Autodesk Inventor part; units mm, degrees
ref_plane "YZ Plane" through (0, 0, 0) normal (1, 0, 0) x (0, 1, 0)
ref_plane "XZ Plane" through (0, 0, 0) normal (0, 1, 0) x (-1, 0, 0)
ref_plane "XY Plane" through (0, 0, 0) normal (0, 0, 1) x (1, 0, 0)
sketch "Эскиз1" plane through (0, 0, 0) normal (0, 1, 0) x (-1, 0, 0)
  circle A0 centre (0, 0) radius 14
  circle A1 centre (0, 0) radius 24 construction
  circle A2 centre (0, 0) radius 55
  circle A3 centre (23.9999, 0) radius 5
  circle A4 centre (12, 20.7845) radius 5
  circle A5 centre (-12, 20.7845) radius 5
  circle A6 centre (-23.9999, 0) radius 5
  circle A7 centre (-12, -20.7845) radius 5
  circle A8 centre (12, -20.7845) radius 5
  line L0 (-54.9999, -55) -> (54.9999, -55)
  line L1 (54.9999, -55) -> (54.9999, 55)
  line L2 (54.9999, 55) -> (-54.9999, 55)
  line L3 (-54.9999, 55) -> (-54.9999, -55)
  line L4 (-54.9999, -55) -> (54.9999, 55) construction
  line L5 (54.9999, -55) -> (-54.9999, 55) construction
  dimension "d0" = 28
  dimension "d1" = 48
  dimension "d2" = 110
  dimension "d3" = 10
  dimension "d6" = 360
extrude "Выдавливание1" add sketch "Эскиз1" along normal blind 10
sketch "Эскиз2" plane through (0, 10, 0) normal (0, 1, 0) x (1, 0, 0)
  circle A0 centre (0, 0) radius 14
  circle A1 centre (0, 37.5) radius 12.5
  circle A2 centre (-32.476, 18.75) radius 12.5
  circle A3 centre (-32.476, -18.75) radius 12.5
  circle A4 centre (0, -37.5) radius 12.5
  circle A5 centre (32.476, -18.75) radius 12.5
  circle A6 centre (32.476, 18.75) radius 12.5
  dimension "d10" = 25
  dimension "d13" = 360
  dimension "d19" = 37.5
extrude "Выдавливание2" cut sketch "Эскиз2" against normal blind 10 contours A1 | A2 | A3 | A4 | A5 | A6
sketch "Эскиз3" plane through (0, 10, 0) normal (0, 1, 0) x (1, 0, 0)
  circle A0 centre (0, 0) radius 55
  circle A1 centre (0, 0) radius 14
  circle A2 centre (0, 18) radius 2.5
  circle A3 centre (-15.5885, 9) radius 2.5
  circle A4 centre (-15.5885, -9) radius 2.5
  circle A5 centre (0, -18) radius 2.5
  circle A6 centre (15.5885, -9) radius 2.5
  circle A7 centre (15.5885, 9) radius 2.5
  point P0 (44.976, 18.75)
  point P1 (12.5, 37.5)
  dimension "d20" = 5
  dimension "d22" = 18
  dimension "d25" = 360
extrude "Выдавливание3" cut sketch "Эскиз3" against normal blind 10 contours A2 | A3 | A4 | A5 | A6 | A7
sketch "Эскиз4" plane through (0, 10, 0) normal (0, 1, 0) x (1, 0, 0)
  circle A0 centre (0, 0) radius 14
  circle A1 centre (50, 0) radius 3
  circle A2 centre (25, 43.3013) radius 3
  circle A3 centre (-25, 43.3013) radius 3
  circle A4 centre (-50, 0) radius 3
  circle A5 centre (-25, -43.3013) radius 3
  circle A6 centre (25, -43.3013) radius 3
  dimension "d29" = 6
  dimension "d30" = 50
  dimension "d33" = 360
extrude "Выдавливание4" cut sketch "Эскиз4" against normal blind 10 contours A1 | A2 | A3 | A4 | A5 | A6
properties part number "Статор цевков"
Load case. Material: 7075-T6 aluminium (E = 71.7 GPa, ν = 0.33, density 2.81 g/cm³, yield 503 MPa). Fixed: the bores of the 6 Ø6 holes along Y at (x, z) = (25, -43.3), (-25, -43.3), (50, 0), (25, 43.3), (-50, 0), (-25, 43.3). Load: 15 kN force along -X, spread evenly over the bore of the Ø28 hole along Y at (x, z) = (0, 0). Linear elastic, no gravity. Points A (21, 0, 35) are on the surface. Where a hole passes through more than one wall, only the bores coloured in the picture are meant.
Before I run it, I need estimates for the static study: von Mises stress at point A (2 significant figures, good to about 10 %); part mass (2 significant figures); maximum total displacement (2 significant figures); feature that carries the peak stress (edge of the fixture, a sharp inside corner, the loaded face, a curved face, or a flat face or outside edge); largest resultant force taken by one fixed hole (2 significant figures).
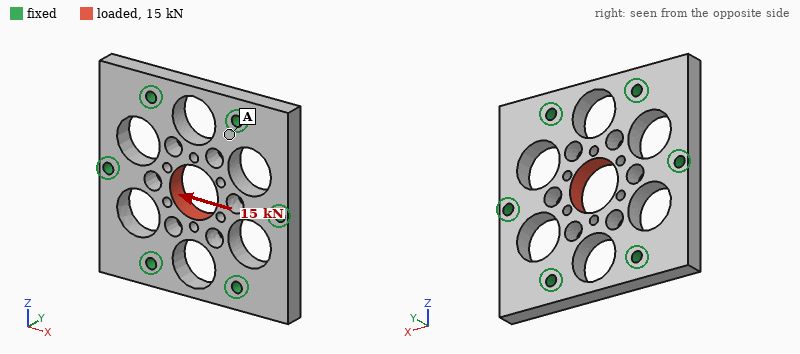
16 MPa
220 g
26 µm
a curved face
4.2 kN
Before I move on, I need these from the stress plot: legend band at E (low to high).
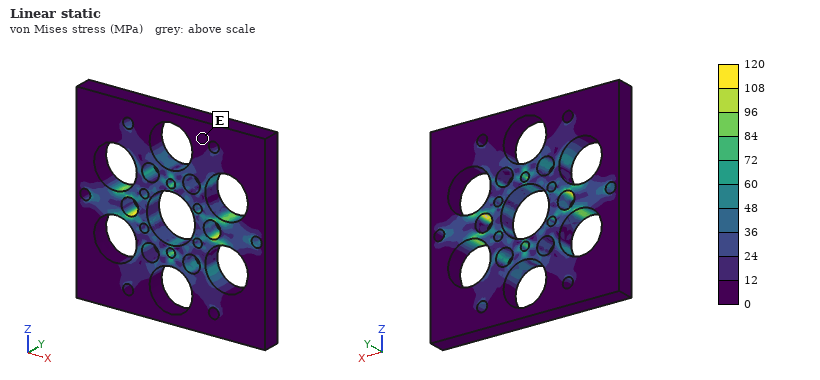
0 to 12 MPa
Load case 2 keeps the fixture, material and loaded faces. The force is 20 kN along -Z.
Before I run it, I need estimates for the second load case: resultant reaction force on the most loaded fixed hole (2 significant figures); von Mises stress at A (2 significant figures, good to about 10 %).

5.0 kN
38 MPa
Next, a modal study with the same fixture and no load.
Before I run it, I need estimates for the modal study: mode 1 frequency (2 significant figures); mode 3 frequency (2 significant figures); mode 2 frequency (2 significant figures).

7700 Hz
9400 Hz
9300 Hz
